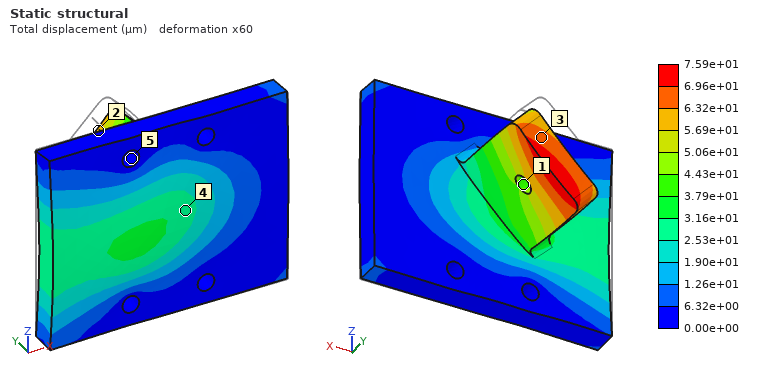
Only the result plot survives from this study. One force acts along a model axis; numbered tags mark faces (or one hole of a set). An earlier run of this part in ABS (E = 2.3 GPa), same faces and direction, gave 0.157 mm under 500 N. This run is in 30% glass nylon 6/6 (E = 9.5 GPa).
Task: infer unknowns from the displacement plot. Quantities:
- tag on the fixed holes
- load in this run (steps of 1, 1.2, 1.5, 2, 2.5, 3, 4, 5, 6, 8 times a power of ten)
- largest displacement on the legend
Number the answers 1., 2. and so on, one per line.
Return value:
1. 5
2. 1 kN
3. 7.59e+01 µm
